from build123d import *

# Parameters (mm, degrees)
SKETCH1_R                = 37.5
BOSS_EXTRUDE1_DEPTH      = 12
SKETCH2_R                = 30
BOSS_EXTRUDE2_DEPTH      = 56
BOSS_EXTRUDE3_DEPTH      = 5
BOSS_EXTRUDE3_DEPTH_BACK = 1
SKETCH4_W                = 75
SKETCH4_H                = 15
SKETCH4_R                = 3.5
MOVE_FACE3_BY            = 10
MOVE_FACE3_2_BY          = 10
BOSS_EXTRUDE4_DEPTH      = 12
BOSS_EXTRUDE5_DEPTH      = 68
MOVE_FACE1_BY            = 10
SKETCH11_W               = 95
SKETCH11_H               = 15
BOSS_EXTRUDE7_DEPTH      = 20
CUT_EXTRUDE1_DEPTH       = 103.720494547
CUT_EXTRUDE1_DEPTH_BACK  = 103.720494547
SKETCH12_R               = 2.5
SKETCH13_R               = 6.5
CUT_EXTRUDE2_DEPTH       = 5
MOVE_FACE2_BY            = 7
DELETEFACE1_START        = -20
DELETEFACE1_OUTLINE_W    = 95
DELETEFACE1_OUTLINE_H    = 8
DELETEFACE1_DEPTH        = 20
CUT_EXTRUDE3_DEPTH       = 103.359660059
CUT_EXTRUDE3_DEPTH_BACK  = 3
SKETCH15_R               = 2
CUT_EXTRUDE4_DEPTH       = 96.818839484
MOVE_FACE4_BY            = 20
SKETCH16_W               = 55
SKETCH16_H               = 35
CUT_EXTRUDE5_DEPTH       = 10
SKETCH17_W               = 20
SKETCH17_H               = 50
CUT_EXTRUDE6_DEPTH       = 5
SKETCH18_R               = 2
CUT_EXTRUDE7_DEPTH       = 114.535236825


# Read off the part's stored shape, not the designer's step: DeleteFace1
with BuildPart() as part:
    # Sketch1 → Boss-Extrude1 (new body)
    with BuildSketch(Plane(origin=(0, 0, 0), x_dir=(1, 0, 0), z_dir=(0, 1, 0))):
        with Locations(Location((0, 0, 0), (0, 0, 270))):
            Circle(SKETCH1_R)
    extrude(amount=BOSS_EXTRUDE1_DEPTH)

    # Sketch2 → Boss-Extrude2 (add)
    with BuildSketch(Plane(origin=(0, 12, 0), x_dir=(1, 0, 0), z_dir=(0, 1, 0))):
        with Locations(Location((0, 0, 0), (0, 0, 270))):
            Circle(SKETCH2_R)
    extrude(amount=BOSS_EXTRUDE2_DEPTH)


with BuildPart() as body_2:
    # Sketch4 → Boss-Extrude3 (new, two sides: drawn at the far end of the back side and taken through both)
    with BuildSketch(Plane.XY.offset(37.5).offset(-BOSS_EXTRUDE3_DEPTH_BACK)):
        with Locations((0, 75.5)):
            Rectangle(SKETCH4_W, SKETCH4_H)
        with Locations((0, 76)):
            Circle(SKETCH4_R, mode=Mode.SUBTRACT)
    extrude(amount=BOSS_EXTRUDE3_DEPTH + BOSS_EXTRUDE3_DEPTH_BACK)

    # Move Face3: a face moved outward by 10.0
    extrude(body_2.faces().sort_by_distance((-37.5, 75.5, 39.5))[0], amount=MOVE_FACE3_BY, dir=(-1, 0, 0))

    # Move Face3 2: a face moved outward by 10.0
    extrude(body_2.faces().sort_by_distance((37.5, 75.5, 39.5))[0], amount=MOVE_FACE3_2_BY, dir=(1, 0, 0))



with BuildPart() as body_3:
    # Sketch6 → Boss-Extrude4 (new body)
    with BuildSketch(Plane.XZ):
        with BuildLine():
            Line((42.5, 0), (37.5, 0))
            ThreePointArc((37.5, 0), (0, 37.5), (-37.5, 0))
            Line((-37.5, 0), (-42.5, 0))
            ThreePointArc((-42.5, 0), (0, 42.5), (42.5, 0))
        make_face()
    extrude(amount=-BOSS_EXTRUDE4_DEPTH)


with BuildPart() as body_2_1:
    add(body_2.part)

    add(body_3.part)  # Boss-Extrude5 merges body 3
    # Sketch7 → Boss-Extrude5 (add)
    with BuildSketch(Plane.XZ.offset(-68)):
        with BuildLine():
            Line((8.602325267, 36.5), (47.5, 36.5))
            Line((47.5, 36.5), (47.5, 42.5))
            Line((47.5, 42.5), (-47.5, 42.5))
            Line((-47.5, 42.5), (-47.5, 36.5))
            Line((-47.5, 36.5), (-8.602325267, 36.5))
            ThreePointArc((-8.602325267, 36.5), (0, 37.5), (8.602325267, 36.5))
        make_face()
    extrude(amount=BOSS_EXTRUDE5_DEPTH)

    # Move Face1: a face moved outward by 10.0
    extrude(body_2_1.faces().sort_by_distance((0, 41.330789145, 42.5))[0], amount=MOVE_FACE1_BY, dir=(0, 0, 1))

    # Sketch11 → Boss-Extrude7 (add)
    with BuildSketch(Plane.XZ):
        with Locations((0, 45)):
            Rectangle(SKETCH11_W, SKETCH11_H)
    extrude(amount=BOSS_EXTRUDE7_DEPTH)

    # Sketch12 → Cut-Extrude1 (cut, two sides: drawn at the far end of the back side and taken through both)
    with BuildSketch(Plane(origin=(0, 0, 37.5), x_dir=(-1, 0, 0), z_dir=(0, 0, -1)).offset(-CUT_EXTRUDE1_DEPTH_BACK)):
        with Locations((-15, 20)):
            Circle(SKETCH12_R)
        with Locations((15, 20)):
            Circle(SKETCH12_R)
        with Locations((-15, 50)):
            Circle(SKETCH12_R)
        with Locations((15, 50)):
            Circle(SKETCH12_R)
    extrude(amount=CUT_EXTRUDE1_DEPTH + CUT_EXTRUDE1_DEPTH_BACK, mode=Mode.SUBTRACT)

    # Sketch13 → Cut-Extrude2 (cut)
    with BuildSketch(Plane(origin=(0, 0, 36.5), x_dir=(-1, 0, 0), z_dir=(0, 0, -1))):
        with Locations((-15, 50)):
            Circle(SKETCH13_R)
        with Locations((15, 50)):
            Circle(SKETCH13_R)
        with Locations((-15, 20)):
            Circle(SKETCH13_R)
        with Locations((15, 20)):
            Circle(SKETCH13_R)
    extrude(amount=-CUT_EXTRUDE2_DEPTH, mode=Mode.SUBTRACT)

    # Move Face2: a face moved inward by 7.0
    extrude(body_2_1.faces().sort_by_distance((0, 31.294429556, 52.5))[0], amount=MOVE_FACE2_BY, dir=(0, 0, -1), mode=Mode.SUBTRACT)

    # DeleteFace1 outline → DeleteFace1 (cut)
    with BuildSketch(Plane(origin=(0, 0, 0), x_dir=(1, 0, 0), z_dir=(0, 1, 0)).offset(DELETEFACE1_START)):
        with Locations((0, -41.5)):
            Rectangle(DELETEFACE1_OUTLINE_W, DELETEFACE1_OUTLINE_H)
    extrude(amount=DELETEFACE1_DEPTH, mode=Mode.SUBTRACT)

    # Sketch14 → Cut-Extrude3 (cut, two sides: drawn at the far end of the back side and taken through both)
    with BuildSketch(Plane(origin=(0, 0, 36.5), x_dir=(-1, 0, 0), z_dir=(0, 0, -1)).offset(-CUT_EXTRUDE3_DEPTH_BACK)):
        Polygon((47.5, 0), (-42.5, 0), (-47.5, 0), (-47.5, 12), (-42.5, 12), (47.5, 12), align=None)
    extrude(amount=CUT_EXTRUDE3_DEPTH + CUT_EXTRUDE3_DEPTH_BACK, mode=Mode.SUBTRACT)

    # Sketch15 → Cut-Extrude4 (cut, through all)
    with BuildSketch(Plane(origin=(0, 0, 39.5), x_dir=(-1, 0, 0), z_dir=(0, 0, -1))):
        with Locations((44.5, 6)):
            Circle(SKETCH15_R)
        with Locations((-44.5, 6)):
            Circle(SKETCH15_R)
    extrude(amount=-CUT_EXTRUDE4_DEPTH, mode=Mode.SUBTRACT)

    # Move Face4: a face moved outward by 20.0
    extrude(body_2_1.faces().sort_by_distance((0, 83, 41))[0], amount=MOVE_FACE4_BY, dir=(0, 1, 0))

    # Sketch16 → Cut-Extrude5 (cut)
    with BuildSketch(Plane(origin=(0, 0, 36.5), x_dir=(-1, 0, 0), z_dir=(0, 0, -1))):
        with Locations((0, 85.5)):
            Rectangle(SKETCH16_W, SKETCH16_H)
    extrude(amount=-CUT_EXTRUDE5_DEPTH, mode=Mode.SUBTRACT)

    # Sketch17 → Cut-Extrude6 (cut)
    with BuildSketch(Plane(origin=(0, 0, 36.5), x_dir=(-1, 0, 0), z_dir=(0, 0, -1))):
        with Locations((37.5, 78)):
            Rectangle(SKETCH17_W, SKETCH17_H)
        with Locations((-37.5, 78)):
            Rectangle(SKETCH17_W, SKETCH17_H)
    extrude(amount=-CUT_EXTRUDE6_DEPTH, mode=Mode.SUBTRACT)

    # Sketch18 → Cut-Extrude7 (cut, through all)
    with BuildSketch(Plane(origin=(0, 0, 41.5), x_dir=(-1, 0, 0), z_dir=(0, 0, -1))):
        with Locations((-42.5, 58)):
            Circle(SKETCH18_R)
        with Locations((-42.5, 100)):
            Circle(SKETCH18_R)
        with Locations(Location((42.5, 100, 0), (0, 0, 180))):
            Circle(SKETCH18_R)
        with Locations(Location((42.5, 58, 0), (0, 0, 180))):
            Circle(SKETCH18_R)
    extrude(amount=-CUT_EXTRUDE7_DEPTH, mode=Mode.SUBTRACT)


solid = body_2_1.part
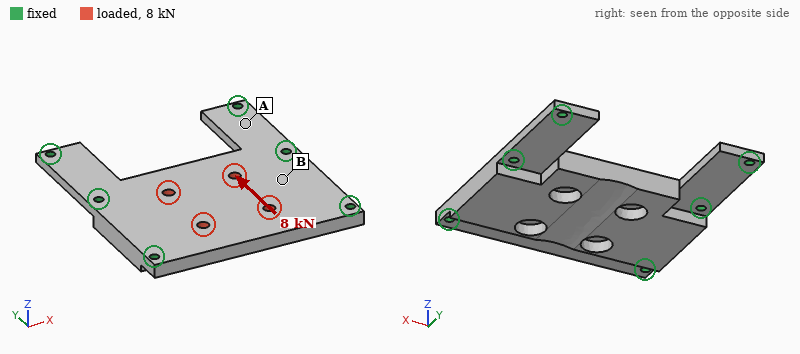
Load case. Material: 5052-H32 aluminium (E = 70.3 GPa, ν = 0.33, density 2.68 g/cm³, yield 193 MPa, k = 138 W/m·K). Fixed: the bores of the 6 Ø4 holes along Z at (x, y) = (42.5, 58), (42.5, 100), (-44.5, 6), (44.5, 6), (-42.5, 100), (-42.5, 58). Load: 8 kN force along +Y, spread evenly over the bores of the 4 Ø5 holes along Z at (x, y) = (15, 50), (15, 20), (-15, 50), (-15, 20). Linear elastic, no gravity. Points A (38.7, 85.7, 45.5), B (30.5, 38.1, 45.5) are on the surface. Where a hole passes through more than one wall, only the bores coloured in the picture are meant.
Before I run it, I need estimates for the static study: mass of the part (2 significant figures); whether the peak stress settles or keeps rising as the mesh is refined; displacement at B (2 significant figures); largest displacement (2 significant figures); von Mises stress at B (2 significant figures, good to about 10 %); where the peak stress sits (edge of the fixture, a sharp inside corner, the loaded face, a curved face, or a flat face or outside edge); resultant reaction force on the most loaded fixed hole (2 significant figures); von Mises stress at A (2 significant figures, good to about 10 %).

140 g
keeps rising
9.1 µm
27 µm
22 MPa
edge of the fixture
2.2 kN
8.7 MPa
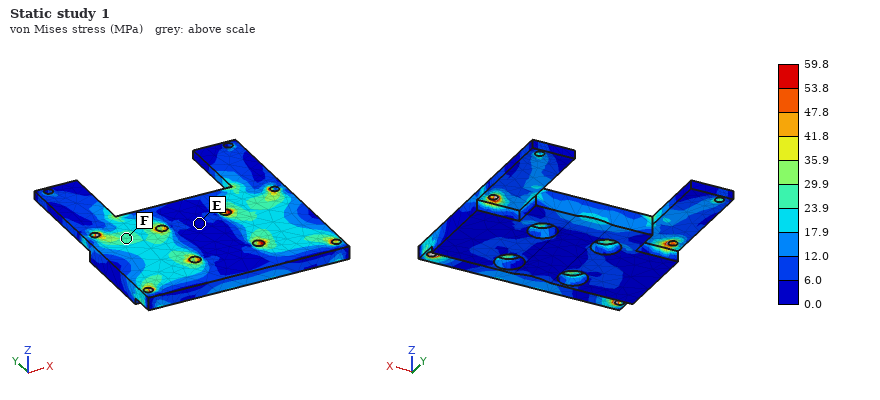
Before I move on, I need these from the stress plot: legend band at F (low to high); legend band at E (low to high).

23.9 to 29.9 MPa
0.0 to 6.0 MPa
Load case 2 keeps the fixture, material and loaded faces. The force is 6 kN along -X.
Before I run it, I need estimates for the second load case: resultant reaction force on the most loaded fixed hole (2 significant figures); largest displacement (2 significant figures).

1.5 kN
9.3 µm
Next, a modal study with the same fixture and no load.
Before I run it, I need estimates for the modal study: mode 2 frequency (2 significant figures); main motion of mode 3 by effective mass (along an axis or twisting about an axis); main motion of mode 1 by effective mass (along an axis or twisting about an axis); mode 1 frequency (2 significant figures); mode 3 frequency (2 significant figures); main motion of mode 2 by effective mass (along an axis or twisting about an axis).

5600 Hz
twisting about Y
along Z
3500 Hz
9000 Hz
twisting about X
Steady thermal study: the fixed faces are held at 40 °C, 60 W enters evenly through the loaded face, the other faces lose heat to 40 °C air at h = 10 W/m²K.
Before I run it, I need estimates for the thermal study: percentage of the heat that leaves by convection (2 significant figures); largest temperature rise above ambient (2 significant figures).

3.9 %
24 K
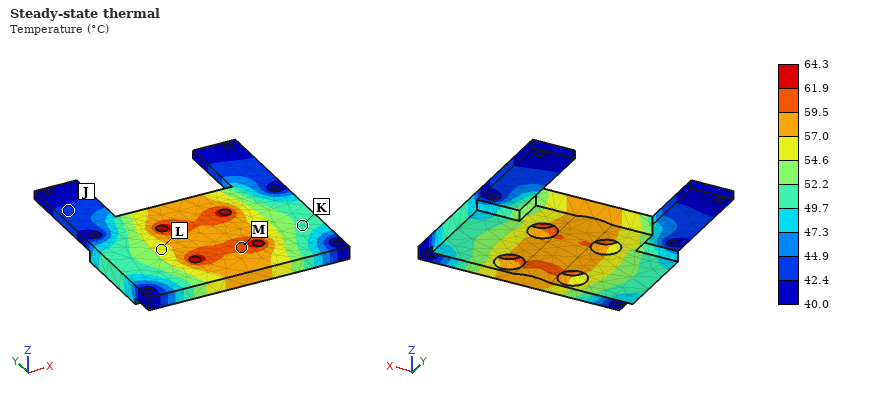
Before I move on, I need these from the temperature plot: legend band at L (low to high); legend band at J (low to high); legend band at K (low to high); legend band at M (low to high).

54.6 to 57.0 °C
42.4 to 44.9 °C
49.7 to 52.2 °C
59.5 to 61.9 °C
